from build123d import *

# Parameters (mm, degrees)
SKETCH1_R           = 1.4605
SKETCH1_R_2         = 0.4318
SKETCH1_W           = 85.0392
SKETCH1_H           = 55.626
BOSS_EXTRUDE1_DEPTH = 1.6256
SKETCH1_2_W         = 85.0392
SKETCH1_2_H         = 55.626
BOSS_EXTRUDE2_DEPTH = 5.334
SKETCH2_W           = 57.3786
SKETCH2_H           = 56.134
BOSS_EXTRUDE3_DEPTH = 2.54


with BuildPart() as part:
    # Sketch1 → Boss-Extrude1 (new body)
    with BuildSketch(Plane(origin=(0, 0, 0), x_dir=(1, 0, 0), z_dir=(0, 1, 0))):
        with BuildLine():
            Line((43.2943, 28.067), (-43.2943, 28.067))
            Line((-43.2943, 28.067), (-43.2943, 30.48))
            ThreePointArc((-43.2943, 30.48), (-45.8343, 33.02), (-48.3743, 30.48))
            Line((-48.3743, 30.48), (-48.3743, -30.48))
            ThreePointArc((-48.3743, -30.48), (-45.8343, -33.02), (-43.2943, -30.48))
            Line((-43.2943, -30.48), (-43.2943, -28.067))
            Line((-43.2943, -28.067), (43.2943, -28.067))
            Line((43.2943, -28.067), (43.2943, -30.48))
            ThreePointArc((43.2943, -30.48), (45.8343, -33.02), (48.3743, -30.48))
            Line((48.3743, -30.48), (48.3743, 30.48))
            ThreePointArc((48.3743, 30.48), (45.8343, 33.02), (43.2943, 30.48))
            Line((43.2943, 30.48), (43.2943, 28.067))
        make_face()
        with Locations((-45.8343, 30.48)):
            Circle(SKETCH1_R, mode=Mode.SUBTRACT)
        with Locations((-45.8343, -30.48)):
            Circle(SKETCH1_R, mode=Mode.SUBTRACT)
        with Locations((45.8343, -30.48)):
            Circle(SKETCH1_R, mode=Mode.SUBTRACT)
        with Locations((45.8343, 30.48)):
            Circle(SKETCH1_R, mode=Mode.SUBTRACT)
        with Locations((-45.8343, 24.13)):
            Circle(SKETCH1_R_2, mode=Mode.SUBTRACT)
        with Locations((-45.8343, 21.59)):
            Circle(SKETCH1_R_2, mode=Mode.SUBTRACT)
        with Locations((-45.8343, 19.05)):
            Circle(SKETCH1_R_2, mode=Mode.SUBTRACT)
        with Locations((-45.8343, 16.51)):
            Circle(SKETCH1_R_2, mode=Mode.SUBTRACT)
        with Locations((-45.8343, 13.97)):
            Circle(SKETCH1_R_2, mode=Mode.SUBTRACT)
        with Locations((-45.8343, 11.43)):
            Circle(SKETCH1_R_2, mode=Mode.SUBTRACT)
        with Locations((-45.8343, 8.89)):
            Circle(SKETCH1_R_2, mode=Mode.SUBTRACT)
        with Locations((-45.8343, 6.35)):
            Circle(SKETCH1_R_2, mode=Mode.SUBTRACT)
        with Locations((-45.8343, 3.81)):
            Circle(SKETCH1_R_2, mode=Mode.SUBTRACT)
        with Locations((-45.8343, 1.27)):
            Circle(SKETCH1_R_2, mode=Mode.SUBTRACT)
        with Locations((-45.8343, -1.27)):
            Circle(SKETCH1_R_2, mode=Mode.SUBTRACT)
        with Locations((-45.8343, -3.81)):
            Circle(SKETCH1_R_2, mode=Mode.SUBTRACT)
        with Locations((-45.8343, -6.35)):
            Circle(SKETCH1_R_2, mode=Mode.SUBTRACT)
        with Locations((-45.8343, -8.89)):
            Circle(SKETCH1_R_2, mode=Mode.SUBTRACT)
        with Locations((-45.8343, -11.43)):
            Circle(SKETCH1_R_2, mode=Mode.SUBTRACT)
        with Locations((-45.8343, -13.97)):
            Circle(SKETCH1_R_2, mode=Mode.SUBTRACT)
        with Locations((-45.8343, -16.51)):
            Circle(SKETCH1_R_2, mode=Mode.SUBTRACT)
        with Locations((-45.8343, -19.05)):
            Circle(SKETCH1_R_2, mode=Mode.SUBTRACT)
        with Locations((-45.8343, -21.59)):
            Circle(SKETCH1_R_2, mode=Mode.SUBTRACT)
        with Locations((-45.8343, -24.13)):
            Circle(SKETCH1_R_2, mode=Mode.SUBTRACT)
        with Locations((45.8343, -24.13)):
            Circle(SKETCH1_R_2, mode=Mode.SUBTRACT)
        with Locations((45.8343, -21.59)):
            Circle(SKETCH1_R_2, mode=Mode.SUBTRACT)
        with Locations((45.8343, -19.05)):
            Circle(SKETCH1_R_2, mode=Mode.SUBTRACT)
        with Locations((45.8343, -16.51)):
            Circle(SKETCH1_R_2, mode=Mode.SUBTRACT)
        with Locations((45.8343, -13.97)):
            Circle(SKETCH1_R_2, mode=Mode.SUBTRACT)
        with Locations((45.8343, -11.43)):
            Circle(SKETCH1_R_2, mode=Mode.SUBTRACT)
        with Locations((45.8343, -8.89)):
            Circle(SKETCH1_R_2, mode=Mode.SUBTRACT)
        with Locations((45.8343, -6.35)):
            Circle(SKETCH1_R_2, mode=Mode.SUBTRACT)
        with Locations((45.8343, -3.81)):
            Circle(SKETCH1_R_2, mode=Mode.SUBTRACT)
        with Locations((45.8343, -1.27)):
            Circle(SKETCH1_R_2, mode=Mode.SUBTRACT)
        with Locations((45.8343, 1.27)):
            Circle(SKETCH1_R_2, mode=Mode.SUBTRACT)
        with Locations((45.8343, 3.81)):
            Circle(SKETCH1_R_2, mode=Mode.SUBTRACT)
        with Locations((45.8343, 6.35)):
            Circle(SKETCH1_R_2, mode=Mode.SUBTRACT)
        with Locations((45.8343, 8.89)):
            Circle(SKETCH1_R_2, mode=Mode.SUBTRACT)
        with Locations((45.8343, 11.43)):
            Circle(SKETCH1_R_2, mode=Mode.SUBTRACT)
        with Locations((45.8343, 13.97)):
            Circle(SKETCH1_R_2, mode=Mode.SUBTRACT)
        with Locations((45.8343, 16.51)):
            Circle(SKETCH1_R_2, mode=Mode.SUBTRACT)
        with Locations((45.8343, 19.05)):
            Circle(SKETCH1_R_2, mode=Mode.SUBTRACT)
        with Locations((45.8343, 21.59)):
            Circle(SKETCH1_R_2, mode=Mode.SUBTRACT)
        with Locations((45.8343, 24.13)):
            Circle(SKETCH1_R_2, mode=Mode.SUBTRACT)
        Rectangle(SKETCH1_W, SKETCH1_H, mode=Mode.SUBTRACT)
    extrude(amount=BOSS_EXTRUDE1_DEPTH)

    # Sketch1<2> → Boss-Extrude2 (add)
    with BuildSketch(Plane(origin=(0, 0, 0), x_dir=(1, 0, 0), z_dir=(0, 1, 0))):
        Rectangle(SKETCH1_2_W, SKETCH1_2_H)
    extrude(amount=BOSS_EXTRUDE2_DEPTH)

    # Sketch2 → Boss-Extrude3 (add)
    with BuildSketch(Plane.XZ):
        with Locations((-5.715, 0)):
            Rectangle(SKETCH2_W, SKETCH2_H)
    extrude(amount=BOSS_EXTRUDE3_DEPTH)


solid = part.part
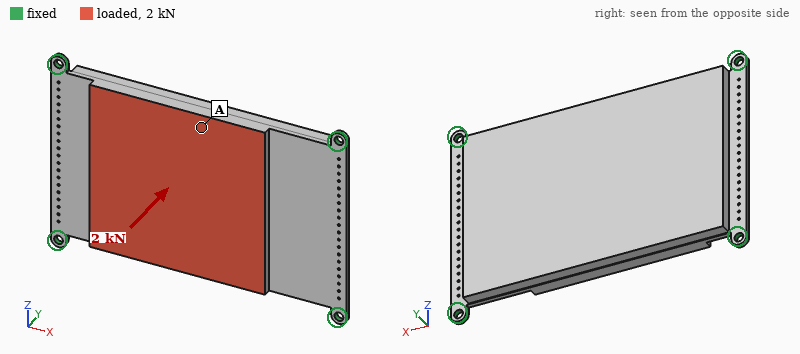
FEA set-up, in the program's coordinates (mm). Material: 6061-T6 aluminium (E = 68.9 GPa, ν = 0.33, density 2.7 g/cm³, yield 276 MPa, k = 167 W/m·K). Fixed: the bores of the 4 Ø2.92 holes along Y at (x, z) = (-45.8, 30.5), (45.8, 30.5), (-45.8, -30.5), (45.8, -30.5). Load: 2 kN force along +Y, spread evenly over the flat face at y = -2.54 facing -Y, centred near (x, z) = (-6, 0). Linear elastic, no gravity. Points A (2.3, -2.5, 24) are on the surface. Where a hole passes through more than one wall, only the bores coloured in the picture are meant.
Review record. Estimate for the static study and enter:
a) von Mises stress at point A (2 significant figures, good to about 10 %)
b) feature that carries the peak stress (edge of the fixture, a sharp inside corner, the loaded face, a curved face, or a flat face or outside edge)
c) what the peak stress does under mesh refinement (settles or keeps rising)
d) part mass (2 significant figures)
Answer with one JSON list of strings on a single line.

["48 MPa", "edge of the fixture", "keeps rising", "93 g"]
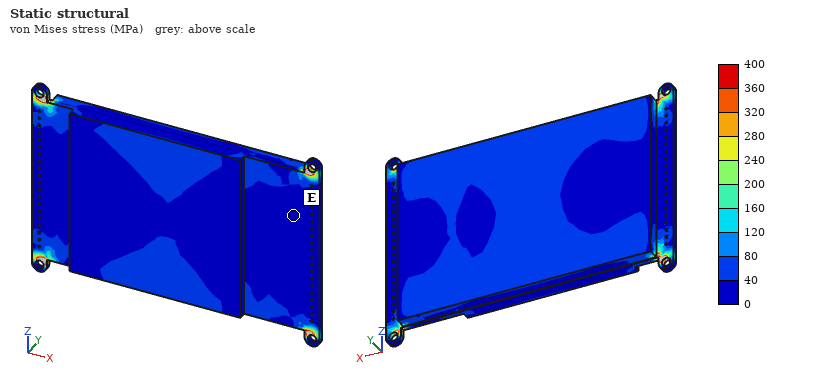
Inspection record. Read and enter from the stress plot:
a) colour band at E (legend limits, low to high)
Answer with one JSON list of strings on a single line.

["0 to 40 MPa"]
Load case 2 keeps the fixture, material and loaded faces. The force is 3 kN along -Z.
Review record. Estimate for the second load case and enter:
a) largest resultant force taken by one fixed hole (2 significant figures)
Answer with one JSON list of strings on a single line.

["900 N"]
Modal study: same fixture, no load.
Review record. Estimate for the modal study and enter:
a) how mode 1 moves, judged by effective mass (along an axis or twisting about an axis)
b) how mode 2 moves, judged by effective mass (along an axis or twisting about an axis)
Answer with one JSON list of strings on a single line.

["along Y", "twisting about X"]
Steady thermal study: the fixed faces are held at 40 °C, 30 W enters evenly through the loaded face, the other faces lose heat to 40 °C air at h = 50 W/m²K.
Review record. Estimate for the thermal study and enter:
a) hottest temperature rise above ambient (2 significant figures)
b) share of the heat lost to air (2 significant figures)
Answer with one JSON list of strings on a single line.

["26 K", "37 %"]
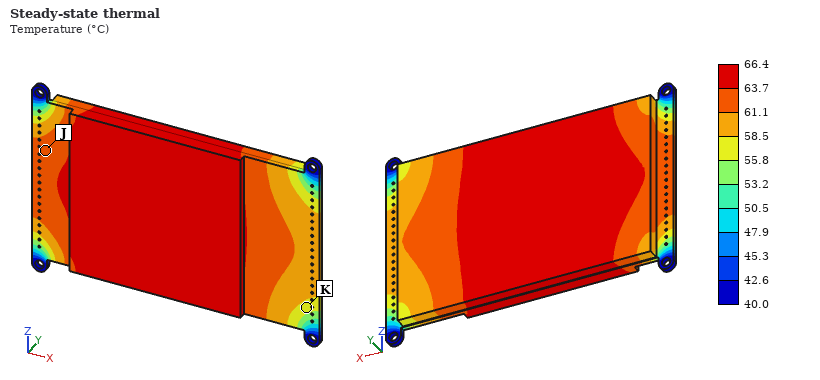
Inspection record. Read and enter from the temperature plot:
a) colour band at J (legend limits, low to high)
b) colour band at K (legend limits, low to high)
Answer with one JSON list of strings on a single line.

["61.1 to 63.7 °C", "55.8 to 58.5 °C"]
